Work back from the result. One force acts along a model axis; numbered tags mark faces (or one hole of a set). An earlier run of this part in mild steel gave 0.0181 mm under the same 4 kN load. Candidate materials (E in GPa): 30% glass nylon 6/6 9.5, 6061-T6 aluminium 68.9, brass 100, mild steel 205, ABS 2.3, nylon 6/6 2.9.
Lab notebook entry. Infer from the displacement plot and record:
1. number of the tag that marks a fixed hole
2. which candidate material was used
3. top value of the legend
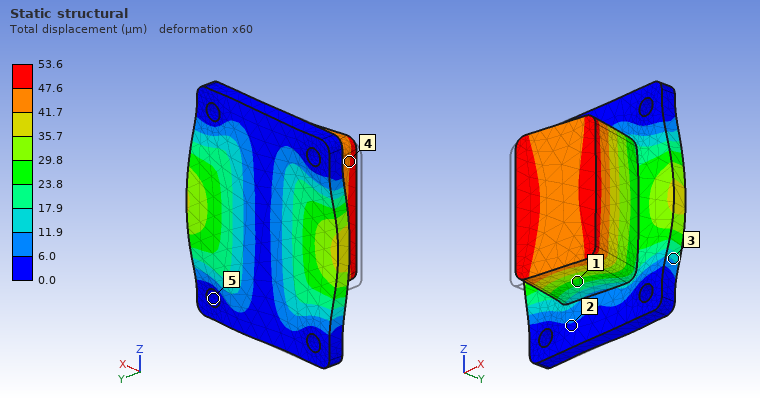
5
6061-T6 aluminium
53.6 µm
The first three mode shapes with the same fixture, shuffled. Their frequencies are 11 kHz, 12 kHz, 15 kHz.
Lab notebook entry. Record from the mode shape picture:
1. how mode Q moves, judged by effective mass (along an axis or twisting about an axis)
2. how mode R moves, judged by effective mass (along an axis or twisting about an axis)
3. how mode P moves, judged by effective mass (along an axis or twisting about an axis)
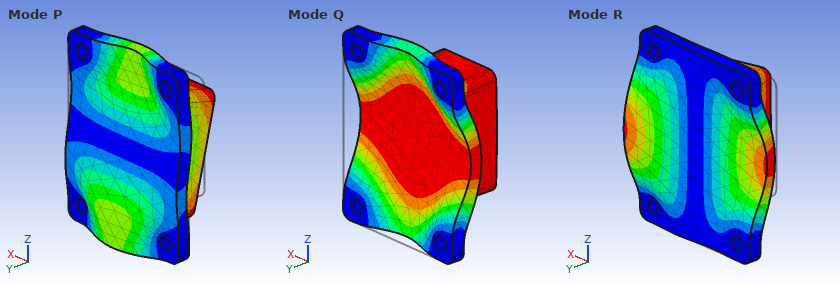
along Y
along X
along Z
